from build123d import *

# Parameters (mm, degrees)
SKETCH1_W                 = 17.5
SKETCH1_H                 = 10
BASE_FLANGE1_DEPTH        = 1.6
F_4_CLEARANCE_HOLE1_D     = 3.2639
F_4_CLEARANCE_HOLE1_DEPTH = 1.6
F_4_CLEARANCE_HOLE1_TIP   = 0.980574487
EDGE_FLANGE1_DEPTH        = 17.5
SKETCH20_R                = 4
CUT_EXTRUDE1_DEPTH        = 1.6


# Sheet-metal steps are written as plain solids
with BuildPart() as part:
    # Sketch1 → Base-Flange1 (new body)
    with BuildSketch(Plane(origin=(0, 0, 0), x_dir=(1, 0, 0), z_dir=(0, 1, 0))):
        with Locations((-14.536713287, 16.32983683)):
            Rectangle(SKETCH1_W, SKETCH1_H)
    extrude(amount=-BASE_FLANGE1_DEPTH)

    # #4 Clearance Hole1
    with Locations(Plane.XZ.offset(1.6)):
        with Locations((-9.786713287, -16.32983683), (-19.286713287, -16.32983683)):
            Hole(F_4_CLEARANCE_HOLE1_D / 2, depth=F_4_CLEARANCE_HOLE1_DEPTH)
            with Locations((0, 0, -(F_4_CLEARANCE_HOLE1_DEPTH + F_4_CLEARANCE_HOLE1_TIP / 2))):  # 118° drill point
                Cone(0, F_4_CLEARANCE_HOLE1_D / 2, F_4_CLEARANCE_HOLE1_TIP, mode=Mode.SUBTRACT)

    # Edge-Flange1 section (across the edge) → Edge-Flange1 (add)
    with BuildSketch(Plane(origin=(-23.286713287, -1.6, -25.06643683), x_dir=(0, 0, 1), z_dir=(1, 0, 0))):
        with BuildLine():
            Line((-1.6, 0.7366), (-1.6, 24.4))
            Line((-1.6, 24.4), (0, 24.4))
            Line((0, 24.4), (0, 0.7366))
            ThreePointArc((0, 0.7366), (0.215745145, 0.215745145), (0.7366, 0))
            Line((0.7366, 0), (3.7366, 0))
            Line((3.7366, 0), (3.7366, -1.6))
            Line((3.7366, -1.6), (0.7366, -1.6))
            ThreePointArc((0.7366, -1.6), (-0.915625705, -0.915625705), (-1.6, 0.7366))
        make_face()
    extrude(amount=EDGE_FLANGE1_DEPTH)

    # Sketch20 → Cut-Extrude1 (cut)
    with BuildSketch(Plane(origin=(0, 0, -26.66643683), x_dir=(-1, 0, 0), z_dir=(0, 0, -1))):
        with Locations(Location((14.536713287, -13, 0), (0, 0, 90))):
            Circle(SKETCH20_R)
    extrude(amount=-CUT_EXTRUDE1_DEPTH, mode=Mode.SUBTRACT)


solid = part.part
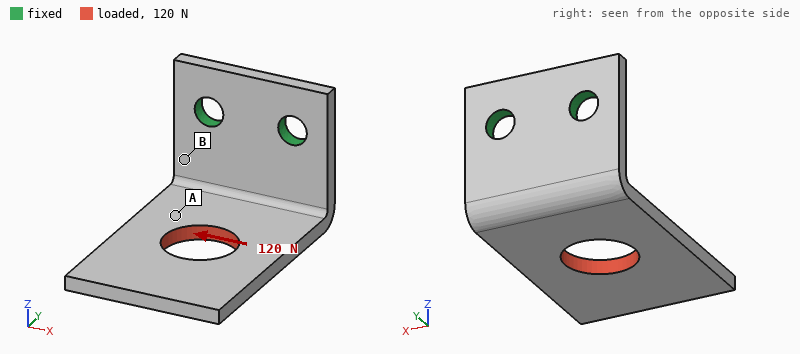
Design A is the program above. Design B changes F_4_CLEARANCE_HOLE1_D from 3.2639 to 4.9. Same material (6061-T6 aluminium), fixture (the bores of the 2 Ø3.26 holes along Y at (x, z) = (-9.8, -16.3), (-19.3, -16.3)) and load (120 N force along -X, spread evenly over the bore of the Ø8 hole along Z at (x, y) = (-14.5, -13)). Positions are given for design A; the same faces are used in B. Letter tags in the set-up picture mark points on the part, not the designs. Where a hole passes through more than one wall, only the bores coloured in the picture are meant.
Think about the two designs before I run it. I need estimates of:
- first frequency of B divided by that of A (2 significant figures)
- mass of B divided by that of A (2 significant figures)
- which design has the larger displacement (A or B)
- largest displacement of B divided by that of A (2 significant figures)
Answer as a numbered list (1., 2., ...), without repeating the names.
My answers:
1. 1.0
2. 0.97
3. A
4. 0.80
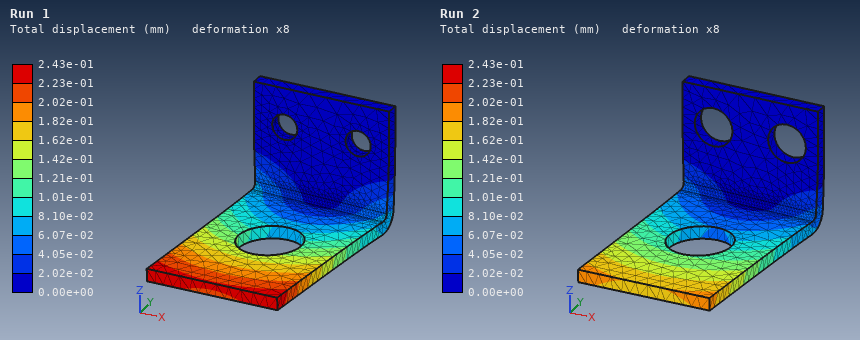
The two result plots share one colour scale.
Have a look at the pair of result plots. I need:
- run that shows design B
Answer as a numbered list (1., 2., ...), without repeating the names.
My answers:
1. Run 2
